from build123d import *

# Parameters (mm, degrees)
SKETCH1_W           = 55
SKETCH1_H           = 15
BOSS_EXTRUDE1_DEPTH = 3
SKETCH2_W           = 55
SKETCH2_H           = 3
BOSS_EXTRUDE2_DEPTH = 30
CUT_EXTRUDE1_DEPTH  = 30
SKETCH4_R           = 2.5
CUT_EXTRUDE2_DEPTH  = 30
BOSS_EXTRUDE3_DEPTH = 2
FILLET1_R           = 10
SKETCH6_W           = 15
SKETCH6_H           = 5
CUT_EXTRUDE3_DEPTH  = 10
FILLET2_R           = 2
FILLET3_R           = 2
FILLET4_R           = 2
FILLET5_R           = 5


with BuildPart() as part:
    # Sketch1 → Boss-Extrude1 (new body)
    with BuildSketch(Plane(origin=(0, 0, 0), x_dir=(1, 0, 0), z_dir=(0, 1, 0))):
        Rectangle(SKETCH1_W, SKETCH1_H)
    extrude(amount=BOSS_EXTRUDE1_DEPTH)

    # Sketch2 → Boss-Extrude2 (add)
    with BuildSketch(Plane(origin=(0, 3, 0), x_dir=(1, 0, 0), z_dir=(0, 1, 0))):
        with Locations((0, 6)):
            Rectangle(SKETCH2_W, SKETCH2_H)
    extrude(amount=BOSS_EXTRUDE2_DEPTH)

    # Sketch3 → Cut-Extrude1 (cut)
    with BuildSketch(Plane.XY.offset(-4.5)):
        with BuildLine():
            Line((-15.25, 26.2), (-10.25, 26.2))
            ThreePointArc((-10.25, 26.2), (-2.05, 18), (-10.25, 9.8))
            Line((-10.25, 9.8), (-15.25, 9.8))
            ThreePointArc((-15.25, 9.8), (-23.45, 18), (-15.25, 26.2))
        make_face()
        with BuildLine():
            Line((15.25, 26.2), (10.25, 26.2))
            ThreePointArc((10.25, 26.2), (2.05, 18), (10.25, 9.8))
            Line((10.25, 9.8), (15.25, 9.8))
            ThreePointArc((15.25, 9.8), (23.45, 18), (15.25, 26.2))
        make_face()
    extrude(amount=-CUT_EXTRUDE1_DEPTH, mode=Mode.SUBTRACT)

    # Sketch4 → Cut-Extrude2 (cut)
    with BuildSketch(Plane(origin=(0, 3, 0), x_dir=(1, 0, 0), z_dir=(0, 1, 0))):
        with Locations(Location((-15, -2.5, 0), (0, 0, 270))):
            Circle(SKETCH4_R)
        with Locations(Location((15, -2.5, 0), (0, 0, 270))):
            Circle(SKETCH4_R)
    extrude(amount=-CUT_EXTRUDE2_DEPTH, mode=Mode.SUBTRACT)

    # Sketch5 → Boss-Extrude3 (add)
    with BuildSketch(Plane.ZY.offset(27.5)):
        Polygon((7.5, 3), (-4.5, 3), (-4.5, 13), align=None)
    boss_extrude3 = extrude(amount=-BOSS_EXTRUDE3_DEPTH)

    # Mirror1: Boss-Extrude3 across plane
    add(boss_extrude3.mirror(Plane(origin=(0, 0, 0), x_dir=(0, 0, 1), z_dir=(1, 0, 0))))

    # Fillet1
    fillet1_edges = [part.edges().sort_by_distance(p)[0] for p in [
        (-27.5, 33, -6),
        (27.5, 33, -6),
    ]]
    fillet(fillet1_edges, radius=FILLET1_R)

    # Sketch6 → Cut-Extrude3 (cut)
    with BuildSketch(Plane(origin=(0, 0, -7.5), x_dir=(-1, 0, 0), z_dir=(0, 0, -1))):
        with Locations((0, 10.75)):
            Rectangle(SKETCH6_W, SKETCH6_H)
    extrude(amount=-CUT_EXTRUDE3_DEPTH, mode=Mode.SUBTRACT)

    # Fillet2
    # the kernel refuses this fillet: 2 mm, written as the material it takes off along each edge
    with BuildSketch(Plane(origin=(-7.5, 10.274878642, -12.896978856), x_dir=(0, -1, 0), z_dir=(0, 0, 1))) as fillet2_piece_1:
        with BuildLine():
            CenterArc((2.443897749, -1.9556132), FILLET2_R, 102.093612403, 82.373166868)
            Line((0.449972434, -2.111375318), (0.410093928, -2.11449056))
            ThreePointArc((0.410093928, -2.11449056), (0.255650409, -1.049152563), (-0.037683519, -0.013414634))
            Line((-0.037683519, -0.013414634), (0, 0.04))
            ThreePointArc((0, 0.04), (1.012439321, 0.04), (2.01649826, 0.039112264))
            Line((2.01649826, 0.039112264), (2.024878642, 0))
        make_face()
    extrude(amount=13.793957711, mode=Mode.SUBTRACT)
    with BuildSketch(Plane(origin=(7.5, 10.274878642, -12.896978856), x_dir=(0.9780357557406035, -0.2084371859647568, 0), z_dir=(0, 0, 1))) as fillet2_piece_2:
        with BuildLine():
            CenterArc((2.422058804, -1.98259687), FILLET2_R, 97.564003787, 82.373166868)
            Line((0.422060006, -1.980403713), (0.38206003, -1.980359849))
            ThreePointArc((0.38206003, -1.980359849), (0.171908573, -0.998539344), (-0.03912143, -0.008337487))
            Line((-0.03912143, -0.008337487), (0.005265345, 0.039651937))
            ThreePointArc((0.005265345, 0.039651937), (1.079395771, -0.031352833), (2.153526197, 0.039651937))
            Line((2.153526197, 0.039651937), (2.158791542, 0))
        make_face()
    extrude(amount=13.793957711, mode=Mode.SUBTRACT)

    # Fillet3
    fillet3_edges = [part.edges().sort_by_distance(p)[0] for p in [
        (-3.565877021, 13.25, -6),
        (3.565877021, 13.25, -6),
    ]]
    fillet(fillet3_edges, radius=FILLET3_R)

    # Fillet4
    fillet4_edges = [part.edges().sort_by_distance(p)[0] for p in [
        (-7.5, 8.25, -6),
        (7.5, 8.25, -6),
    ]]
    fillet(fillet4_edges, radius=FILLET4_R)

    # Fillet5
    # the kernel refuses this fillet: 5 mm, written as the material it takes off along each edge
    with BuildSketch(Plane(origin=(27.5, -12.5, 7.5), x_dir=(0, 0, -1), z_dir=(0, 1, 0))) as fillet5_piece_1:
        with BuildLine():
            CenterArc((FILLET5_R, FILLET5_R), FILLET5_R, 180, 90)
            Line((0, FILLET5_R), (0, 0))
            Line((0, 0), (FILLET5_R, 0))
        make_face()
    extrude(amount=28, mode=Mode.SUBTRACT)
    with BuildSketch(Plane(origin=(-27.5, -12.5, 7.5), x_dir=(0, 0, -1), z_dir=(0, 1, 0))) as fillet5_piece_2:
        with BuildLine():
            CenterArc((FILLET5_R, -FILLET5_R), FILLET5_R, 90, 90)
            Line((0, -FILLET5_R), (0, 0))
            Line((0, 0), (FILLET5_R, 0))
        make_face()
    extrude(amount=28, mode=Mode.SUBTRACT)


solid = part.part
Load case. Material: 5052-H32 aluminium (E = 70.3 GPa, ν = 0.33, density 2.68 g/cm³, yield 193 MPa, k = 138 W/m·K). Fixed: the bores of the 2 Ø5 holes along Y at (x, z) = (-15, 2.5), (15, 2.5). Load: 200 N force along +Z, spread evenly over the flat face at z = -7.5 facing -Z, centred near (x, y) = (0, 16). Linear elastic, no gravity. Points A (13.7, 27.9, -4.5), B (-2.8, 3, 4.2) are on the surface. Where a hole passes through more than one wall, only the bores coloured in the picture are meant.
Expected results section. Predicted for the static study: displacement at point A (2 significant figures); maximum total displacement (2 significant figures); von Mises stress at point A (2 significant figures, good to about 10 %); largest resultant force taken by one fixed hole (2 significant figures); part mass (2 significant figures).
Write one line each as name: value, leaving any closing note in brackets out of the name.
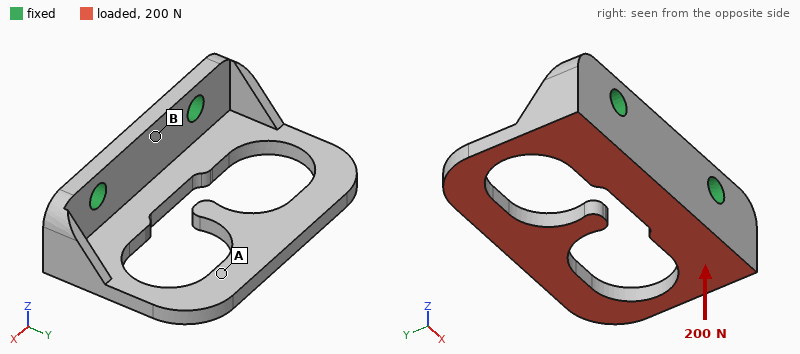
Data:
displacement at point A: 0.23 mm
maximum total displacement: 0.31 mm
von Mises stress at point A: 19 MPa
largest resultant force taken by one fixed hole: 100 N
part mass: 15 g
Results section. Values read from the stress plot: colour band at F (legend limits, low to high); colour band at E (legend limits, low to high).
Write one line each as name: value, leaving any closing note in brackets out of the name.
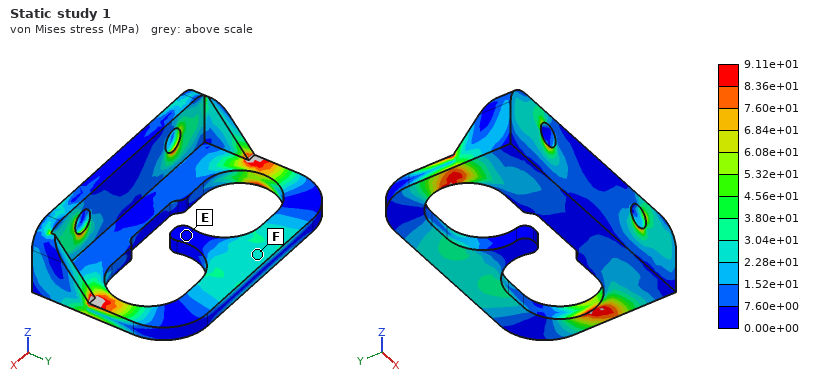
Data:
colour band at F: 2.28e+01 to 3.04e+01 MPa
colour band at E: 0.00e+00 to 7.60e+00 MPa
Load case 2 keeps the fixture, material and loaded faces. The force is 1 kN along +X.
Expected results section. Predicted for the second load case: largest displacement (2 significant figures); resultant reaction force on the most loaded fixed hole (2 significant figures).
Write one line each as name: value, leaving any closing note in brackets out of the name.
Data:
largest displacement: 0.14 mm
resultant reaction force on the most loaded fixed hole: 680 N
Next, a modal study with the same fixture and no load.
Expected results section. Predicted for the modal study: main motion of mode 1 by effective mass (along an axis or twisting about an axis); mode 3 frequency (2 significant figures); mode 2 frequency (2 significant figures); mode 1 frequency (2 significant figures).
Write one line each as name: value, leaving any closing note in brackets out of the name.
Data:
main motion of mode 1 by effective mass: along Z
mode 3 frequency: 4700 Hz
mode 2 frequency: 3600 Hz
mode 1 frequency: 1600 Hz
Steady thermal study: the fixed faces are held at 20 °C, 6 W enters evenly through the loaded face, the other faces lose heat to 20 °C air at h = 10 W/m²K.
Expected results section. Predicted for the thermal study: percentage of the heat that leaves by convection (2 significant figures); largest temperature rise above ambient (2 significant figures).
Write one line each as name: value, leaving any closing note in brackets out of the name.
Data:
percentage of the heat that leaves by convection: 3.8 %
largest temperature rise above ambient: 21 K
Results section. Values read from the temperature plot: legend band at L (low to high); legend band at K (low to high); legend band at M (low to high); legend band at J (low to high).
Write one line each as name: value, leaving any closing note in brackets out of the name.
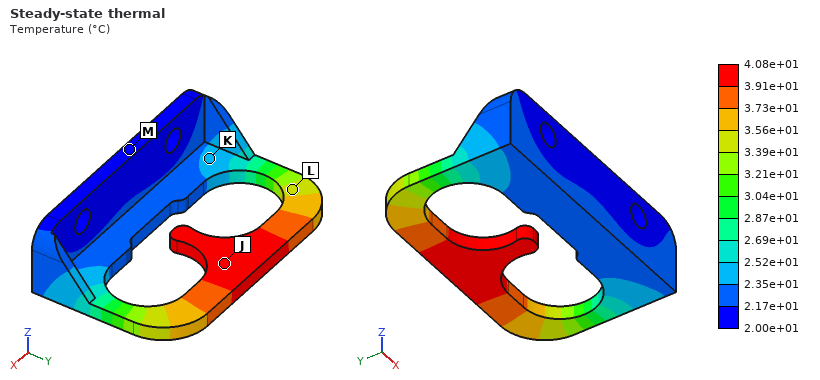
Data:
legend band at L: 3.39e+01 to 3.56e+01 °C
legend band at K: 2.35e+01 to 2.52e+01 °C
legend band at M: 2.00e+01 to 2.17e+01 °C
legend band at J: 3.91e+01 to 4.08e+01 °C
